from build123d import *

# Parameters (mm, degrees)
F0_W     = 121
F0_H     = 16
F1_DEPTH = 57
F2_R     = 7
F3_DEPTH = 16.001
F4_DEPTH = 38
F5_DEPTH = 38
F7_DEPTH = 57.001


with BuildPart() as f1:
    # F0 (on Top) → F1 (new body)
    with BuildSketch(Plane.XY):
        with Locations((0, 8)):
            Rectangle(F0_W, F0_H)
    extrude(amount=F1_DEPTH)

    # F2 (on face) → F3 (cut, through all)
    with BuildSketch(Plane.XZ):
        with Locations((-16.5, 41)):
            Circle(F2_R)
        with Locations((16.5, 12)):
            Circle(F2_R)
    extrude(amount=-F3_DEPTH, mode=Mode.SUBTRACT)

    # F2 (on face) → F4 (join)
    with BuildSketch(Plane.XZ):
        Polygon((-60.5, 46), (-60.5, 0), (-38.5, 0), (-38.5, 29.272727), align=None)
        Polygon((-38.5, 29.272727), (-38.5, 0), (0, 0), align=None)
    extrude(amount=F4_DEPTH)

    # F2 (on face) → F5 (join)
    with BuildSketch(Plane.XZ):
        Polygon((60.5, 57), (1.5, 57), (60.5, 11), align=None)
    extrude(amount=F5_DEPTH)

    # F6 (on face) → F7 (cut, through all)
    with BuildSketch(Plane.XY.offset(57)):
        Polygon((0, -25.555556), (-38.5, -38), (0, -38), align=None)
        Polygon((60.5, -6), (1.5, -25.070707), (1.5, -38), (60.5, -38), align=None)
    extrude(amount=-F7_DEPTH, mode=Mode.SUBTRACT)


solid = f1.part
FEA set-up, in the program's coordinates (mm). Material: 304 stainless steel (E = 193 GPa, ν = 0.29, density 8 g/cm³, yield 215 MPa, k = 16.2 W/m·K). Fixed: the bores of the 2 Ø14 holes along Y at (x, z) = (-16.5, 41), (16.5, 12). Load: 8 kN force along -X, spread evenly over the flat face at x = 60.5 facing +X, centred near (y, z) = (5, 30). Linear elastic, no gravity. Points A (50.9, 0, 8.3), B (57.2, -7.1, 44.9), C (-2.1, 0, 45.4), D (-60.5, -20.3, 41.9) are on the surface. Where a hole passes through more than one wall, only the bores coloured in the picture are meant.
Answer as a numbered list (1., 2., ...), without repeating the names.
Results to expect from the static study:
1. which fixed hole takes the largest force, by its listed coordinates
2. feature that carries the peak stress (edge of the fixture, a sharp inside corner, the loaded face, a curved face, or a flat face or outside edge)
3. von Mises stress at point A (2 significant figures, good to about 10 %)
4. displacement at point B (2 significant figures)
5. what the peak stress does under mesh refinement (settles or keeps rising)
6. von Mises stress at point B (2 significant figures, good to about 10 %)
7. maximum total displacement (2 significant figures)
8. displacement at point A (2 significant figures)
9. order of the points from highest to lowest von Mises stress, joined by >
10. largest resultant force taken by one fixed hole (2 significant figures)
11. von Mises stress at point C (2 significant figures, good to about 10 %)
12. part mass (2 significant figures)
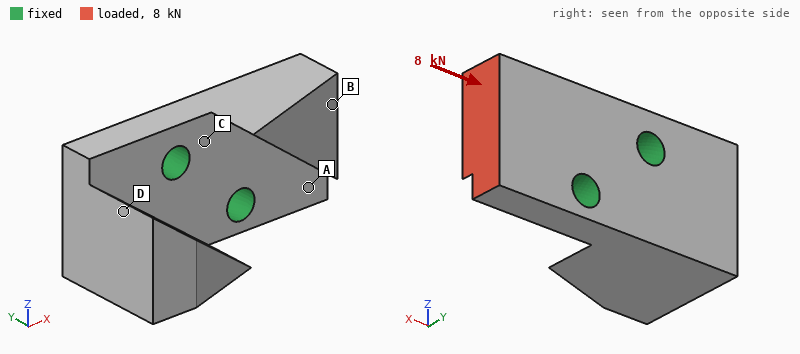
1. (16.5, 12)
2. edge of the fixture
3. 9.9 MPa
4. 5.3 µm
5. keeps rising
6. 4.7 MPa
7. 6.2 µm
8. 2.3 µm
9. C > A > B > D
10. 4.5 kN
11. 14 MPa
12. 1.4 kg
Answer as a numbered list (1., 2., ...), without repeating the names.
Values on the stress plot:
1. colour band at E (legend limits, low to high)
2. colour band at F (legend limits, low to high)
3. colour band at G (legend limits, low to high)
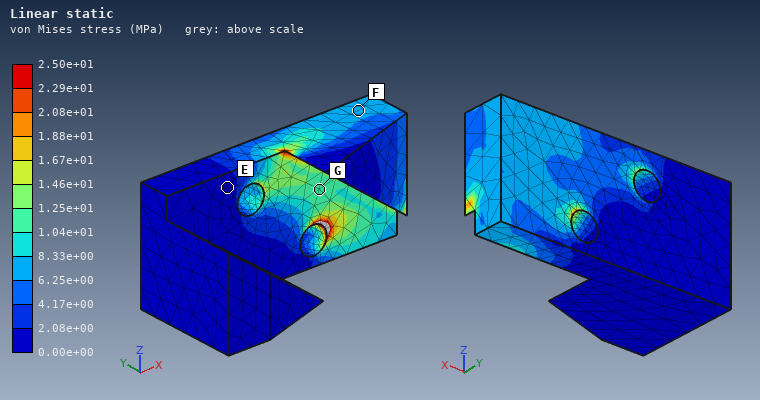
1. 0.00e+00 to 2.08e+00 MPa
2. 6.25e+00 to 8.33e+00 MPa
3. 1.04e+01 to 1.25e+01 MPa
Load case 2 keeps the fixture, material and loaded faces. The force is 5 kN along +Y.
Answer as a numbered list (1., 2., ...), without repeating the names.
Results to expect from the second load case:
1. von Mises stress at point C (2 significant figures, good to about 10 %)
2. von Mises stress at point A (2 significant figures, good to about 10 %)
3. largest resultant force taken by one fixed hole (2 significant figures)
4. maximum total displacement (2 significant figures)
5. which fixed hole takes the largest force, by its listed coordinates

1. 37 MPa
2. 17 MPa
3. 6.1 kN
4. 56 µm
5. (16.5, 12)
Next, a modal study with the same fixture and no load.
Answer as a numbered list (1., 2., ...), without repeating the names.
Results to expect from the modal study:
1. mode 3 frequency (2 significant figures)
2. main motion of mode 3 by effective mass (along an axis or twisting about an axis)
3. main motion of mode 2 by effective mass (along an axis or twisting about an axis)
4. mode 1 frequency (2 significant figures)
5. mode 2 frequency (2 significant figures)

1. 4500 Hz
2. along Z
3. along Y
4. 2300 Hz
5. 3800 Hz
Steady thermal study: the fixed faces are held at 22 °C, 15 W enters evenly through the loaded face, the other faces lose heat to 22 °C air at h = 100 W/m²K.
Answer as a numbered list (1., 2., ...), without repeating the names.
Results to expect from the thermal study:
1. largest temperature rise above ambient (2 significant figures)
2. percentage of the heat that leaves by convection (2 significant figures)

1. 26 K
2. 63 %
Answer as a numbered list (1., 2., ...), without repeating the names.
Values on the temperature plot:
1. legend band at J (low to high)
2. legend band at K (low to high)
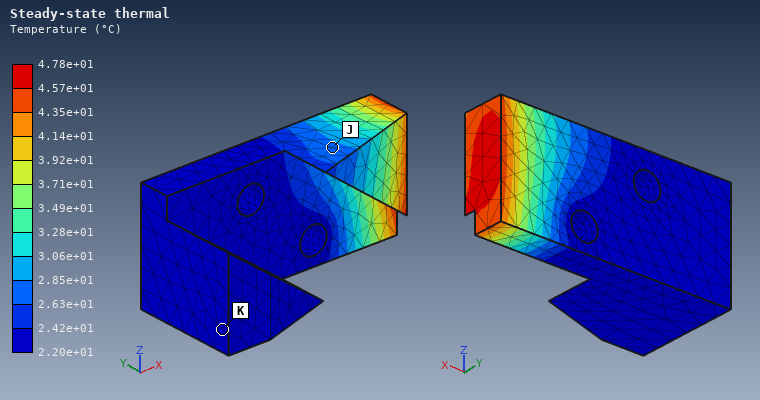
1. 2.63e+01 to 2.85e+01 °C
2. 2.20e+01 to 2.42e+01 °C
